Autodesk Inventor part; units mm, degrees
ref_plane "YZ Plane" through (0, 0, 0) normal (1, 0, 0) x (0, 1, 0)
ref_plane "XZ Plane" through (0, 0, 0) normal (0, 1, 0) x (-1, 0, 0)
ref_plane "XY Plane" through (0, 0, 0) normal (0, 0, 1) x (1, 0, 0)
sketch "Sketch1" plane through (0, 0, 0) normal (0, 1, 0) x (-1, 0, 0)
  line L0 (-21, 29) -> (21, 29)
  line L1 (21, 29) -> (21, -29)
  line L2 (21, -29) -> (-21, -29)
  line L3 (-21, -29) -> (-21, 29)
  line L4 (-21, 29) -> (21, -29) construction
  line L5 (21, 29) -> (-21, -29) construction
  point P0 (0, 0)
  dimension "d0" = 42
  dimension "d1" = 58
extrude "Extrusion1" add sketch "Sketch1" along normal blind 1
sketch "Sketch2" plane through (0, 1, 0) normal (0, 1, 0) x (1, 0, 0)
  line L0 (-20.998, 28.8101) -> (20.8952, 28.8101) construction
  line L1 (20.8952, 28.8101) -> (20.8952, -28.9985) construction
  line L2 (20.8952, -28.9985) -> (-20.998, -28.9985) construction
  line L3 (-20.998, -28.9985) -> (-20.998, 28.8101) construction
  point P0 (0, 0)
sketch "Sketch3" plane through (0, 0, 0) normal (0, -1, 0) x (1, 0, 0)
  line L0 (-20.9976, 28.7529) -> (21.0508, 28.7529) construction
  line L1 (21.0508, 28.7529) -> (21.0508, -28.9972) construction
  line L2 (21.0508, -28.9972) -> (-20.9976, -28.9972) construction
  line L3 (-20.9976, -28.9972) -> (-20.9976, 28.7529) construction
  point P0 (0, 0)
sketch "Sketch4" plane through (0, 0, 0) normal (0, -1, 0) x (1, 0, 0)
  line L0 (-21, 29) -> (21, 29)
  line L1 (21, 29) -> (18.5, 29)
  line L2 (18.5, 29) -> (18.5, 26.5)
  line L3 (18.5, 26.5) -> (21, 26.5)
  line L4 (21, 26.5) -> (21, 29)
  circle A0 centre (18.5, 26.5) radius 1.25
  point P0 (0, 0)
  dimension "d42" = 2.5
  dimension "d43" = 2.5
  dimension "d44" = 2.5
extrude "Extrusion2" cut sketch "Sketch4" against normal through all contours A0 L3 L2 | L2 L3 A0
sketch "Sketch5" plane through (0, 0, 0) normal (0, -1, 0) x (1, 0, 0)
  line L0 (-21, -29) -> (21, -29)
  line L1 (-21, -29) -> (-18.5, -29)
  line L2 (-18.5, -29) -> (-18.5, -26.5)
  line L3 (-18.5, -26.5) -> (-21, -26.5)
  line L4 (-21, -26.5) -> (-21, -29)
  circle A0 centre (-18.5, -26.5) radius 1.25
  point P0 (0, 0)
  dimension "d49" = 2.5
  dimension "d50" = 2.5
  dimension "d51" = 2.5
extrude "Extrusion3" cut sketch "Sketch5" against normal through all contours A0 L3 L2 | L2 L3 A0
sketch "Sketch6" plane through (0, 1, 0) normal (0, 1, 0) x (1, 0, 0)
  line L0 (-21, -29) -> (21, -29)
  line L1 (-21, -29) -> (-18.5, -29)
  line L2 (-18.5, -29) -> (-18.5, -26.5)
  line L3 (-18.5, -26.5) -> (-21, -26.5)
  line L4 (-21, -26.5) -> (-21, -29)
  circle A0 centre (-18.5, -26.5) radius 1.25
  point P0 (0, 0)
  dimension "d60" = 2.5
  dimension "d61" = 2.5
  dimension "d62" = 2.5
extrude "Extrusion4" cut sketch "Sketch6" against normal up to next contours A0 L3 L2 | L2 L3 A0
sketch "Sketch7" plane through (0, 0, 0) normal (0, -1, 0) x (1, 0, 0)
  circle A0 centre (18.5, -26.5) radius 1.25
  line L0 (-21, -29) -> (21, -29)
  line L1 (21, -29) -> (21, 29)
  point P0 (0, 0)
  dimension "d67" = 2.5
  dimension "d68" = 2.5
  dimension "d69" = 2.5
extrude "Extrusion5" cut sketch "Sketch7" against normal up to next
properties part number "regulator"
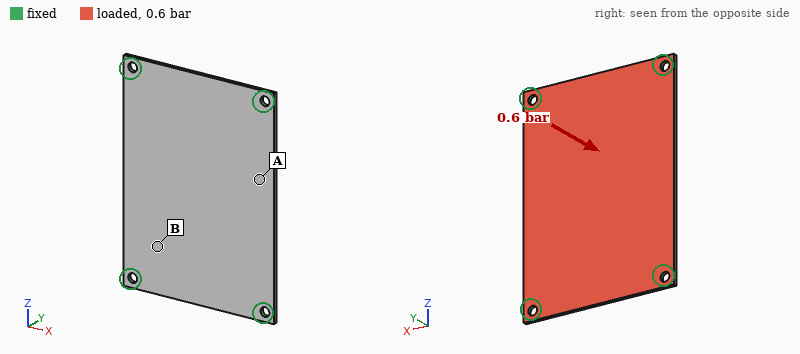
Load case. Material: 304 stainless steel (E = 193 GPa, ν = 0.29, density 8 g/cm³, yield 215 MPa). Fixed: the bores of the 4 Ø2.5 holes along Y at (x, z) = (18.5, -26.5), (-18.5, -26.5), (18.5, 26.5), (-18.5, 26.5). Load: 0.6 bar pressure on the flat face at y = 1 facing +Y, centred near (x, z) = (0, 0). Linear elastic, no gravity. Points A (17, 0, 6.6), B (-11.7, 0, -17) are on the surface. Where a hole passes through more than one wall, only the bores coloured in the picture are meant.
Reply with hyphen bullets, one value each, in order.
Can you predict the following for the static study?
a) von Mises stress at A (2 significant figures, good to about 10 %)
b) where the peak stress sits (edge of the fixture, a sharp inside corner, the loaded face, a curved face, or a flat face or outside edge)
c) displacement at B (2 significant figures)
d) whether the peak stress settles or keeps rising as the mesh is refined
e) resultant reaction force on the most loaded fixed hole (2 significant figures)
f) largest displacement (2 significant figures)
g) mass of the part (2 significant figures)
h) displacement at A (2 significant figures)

- 46 MPa
- edge of the fixture
- 0.054 mm
- keeps rising
- 36 N
- 0.12 mm
- 19 g
- 0.095 mm
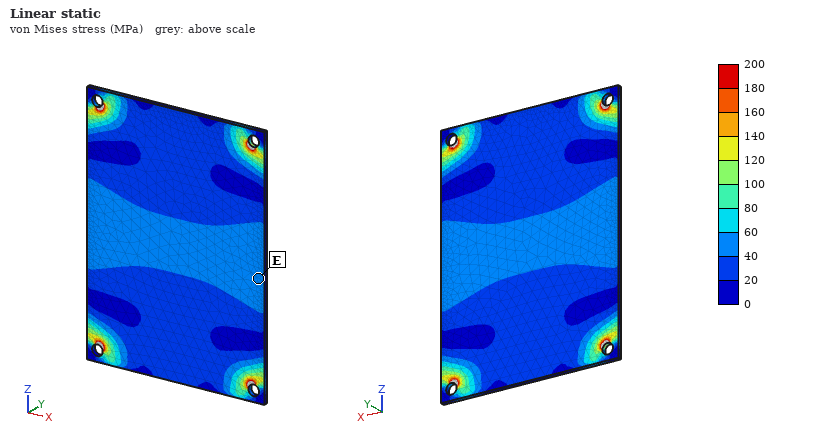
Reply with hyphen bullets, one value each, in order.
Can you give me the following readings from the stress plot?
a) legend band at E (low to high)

- 40 to 60 MPa
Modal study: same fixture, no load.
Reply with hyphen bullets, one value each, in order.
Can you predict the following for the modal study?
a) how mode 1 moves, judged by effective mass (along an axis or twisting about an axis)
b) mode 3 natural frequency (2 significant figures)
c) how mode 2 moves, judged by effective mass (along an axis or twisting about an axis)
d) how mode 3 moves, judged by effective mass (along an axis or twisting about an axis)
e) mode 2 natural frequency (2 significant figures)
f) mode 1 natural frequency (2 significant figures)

- along Y
- 3400 Hz
- twisting about Z
- twisting about X
- 2400 Hz
- 1500 Hz
